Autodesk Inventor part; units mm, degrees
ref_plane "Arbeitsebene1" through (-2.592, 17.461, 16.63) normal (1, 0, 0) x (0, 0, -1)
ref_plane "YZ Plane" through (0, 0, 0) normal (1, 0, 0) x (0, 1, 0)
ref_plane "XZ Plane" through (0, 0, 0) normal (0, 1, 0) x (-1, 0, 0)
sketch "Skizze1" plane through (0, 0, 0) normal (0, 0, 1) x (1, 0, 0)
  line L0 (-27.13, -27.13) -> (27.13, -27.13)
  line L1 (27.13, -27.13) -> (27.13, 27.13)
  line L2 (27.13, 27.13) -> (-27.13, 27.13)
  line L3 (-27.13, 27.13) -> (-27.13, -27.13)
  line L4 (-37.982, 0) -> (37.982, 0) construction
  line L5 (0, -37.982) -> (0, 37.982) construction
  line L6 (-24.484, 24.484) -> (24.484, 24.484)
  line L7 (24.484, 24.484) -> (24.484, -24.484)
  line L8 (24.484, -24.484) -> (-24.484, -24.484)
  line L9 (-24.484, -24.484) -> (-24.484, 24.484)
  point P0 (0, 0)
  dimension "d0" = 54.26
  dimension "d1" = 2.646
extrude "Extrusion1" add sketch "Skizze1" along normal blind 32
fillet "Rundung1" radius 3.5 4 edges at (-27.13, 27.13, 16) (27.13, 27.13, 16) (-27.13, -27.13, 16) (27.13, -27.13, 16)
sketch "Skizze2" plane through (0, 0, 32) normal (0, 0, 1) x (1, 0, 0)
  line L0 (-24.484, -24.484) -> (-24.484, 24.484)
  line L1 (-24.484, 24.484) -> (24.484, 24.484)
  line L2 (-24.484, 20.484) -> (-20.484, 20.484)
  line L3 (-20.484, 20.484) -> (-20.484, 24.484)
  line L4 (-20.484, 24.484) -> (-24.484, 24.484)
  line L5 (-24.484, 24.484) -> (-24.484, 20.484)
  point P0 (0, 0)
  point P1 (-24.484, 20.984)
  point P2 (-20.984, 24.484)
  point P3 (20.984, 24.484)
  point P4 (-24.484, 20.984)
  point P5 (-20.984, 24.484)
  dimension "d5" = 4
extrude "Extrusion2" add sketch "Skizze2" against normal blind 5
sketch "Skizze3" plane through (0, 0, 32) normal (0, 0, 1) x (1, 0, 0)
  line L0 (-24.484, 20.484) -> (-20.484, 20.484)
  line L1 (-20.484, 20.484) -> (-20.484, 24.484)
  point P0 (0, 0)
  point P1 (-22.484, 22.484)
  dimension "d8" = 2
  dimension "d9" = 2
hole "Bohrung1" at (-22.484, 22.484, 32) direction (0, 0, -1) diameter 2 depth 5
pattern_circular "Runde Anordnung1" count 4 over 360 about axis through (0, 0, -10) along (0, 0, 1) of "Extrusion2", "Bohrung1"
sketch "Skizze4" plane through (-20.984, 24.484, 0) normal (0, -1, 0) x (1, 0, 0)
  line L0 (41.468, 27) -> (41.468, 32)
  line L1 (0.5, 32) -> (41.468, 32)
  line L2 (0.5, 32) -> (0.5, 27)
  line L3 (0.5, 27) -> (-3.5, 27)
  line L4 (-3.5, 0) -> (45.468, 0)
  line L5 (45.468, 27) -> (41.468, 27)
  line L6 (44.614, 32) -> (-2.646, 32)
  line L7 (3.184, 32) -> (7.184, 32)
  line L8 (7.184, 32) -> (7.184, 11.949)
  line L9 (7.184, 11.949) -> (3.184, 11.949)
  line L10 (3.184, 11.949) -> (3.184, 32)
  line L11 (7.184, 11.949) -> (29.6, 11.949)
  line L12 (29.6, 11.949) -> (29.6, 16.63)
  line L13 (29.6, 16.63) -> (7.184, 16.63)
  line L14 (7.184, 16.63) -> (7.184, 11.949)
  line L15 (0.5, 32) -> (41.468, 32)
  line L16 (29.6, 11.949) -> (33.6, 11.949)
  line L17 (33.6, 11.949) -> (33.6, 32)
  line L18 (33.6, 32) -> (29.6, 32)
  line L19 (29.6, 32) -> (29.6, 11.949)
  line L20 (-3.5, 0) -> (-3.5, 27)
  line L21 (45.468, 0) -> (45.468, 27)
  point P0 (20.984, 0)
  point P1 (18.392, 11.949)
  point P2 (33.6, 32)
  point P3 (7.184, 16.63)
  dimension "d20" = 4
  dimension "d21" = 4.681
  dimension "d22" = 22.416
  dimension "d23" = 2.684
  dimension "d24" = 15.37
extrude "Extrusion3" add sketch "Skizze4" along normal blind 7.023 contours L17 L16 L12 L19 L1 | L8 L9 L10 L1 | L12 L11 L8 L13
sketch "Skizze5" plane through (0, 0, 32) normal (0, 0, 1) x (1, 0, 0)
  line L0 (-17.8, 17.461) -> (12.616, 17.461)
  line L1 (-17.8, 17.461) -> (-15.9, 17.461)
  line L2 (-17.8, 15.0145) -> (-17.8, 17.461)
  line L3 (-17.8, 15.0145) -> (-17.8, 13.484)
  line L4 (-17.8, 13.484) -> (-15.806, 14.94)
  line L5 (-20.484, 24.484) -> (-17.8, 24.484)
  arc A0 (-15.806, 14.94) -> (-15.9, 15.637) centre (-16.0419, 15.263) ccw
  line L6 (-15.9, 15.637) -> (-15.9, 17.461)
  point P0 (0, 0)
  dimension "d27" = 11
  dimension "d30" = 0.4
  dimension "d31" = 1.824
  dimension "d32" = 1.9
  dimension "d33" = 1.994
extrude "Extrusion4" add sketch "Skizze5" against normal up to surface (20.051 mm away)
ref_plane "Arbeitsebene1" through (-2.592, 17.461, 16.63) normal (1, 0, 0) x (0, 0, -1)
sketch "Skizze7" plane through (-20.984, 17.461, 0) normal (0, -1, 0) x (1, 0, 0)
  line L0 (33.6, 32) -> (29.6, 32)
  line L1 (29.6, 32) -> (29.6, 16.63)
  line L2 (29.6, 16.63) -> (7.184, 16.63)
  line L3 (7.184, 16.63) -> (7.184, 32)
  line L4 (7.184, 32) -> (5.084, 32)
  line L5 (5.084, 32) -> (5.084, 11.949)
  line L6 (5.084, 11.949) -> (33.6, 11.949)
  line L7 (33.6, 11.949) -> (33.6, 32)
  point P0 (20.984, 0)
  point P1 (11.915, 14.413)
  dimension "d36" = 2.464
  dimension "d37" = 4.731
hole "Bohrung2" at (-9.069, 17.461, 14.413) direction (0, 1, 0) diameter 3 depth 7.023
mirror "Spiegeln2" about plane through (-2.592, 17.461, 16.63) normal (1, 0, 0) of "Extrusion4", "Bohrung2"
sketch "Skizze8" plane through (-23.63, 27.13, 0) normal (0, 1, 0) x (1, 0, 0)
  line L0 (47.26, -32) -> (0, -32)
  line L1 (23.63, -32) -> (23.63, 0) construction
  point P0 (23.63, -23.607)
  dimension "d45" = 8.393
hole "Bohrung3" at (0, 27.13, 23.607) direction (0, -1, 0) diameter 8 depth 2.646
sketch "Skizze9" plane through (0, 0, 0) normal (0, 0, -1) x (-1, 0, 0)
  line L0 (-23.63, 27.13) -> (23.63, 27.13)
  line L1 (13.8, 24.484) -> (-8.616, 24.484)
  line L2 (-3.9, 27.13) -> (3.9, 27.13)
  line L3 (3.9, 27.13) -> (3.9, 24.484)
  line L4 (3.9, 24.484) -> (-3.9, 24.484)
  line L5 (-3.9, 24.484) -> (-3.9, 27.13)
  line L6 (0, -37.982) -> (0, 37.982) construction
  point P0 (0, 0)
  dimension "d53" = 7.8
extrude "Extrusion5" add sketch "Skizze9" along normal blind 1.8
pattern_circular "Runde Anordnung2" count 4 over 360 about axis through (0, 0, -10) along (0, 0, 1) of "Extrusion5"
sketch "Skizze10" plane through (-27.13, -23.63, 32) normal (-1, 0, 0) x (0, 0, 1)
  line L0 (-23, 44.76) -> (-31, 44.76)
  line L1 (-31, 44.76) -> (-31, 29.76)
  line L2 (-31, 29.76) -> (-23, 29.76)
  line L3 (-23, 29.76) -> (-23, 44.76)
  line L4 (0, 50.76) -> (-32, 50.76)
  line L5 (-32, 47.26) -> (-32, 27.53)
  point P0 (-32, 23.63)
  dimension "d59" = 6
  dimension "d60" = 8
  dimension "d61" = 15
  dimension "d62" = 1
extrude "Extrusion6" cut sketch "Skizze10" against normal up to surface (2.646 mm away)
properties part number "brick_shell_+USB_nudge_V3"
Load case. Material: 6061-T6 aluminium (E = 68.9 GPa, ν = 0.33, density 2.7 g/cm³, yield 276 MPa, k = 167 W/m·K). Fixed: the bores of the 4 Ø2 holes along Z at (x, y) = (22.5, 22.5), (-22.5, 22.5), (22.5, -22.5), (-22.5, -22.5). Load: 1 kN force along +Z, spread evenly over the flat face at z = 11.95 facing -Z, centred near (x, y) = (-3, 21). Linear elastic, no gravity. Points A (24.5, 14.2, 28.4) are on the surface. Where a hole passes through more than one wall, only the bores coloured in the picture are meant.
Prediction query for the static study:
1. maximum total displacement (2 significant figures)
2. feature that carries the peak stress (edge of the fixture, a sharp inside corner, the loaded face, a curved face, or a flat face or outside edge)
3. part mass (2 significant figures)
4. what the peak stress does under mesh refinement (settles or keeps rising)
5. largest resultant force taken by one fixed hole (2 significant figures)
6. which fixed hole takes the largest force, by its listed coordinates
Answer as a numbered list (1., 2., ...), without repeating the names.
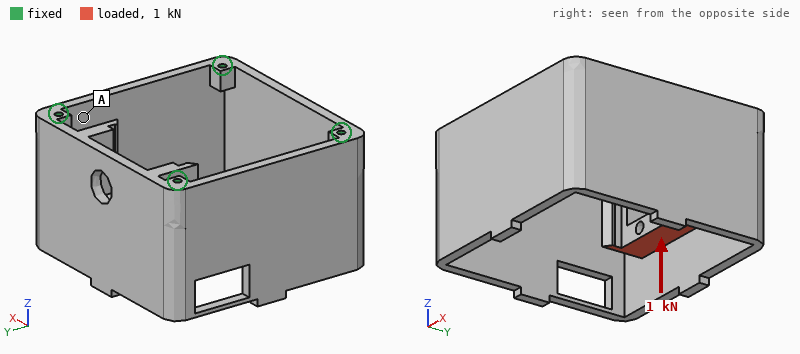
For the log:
1. 59 µm
2. edge of the fixture
3. 52 g
4. keeps rising
5. 540 N
6. (-22.5, 22.5)
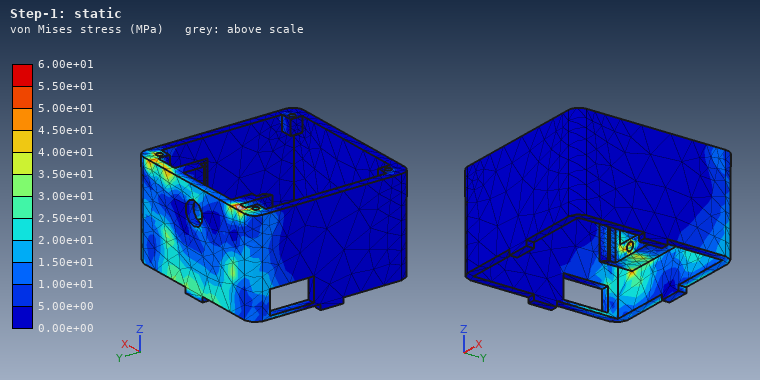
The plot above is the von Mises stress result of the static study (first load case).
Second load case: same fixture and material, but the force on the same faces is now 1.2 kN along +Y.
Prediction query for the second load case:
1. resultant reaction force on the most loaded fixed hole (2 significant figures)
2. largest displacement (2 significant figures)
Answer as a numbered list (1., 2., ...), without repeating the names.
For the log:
1. 490 N
2. 0.23 mm
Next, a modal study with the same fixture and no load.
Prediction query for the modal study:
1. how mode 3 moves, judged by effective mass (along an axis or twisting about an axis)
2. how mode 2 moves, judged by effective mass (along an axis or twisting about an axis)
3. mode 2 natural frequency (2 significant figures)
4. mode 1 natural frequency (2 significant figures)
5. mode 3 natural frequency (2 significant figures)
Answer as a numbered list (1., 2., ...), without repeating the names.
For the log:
1. along Y
2. along X
3. 4300 Hz
4. 3400 Hz
5. 4600 Hz
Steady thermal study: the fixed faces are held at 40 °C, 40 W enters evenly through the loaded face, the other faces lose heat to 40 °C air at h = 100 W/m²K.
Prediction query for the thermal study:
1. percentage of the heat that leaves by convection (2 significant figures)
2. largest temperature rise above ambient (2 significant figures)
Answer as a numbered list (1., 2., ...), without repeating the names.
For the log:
1. 35 %
2. 38 K
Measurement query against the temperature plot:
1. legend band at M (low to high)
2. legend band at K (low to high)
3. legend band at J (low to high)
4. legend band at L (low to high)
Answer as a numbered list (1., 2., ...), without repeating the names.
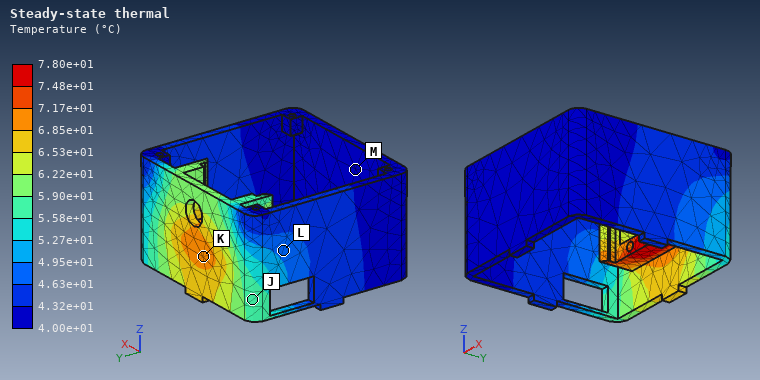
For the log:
1. 4.00e+01 to 4.32e+01 °C
2. 6.85e+01 to 7.17e+01 °C
3. 5.58e+01 to 5.90e+01 °C
4. 4.63e+01 to 4.95e+01 °C
